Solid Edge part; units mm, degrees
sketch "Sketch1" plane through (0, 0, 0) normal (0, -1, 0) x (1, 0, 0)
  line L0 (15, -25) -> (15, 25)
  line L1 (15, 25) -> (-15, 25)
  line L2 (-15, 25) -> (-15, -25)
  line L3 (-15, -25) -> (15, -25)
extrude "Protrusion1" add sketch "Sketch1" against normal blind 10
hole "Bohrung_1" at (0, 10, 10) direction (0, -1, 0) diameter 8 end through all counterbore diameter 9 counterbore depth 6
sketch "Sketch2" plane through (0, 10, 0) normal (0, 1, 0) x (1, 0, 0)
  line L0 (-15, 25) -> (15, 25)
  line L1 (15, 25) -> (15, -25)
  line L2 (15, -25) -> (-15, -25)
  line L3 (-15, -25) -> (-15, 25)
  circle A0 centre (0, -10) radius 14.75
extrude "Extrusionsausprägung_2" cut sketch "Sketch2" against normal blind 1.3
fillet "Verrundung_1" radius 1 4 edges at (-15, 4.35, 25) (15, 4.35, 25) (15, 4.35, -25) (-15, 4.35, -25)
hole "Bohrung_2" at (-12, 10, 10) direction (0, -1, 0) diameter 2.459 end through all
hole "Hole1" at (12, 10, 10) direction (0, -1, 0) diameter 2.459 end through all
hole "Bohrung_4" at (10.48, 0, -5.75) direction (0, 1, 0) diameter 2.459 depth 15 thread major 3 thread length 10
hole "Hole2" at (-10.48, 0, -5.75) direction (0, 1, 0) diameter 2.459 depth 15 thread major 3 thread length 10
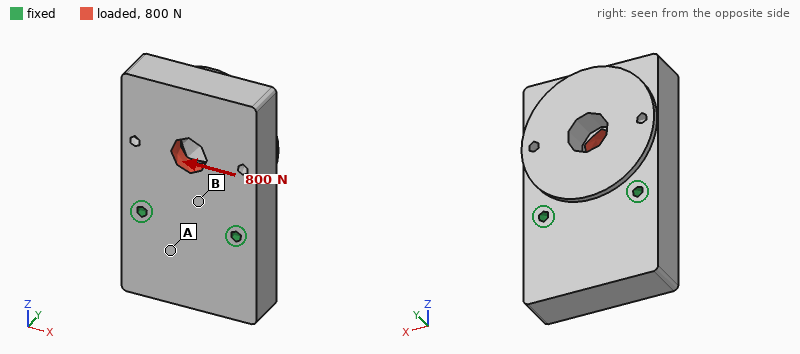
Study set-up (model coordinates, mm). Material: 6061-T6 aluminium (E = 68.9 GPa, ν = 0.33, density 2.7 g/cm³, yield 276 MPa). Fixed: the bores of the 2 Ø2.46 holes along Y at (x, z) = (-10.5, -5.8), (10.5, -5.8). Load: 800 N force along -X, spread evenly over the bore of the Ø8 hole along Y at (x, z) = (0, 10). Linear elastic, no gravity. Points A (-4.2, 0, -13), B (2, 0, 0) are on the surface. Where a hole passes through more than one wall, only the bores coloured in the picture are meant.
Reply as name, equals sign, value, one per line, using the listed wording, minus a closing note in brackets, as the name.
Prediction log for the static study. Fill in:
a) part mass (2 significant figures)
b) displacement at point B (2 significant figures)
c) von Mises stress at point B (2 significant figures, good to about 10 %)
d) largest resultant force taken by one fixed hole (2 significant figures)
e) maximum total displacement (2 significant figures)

part mass = 36 g
displacement at point B = 1.3 µm
von Mises stress at point B = 10 MPa
largest resultant force taken by one fixed hole = 700 N
maximum total displacement = 6.8 µm
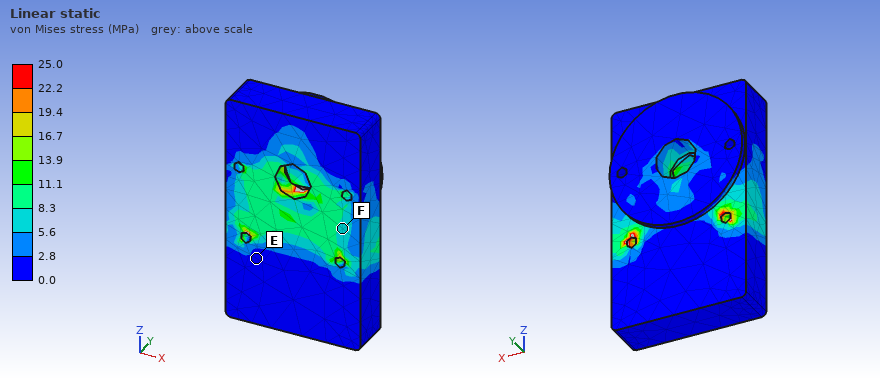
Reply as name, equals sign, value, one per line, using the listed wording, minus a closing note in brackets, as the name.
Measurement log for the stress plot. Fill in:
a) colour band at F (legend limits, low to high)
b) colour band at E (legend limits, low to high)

colour band at F = 5.6 to 8.3 MPa
colour band at E = 0.0 to 2.8 MPa
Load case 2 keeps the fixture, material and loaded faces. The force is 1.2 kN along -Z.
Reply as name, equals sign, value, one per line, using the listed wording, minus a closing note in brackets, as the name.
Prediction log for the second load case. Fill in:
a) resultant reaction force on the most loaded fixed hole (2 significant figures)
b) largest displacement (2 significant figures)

resultant reaction force on the most loaded fixed hole = 610 N
largest displacement = 11 µm
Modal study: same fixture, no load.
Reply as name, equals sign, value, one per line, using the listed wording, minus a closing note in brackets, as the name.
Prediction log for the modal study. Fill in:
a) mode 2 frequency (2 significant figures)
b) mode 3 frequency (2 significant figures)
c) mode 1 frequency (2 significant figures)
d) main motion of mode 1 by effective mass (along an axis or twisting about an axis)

mode 2 frequency = 15 kHz
mode 3 frequency = 15 kHz
mode 1 frequency = 6200 Hz
main motion of mode 1 by effective mass = along Y
